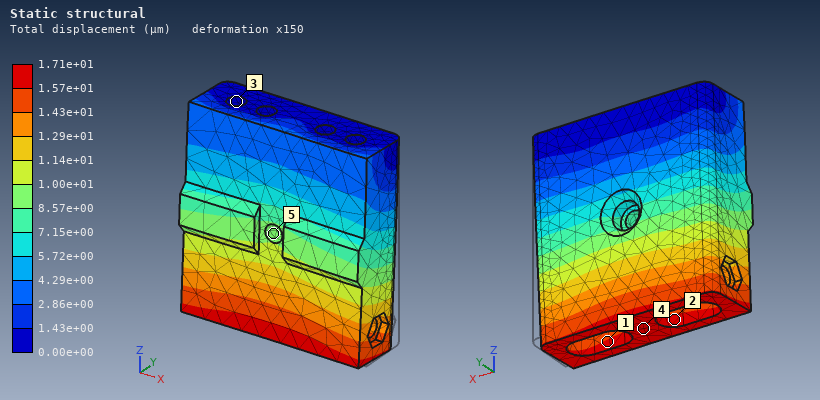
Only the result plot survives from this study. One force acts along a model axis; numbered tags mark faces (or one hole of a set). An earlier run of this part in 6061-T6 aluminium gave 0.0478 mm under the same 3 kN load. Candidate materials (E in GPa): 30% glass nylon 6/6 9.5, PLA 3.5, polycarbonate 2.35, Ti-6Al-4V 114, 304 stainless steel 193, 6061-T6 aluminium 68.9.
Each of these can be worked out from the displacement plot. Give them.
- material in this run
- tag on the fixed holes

304 stainless steel
3
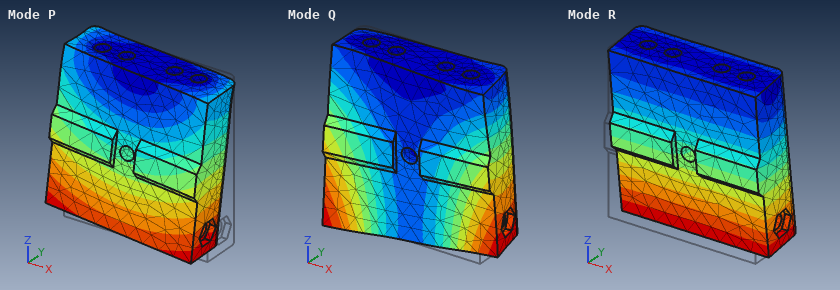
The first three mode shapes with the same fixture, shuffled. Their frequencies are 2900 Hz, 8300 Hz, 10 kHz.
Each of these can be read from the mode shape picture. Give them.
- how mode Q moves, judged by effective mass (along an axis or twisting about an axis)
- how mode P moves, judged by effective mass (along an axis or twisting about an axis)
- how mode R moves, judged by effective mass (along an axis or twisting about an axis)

twisting about Z
along X
along Y
